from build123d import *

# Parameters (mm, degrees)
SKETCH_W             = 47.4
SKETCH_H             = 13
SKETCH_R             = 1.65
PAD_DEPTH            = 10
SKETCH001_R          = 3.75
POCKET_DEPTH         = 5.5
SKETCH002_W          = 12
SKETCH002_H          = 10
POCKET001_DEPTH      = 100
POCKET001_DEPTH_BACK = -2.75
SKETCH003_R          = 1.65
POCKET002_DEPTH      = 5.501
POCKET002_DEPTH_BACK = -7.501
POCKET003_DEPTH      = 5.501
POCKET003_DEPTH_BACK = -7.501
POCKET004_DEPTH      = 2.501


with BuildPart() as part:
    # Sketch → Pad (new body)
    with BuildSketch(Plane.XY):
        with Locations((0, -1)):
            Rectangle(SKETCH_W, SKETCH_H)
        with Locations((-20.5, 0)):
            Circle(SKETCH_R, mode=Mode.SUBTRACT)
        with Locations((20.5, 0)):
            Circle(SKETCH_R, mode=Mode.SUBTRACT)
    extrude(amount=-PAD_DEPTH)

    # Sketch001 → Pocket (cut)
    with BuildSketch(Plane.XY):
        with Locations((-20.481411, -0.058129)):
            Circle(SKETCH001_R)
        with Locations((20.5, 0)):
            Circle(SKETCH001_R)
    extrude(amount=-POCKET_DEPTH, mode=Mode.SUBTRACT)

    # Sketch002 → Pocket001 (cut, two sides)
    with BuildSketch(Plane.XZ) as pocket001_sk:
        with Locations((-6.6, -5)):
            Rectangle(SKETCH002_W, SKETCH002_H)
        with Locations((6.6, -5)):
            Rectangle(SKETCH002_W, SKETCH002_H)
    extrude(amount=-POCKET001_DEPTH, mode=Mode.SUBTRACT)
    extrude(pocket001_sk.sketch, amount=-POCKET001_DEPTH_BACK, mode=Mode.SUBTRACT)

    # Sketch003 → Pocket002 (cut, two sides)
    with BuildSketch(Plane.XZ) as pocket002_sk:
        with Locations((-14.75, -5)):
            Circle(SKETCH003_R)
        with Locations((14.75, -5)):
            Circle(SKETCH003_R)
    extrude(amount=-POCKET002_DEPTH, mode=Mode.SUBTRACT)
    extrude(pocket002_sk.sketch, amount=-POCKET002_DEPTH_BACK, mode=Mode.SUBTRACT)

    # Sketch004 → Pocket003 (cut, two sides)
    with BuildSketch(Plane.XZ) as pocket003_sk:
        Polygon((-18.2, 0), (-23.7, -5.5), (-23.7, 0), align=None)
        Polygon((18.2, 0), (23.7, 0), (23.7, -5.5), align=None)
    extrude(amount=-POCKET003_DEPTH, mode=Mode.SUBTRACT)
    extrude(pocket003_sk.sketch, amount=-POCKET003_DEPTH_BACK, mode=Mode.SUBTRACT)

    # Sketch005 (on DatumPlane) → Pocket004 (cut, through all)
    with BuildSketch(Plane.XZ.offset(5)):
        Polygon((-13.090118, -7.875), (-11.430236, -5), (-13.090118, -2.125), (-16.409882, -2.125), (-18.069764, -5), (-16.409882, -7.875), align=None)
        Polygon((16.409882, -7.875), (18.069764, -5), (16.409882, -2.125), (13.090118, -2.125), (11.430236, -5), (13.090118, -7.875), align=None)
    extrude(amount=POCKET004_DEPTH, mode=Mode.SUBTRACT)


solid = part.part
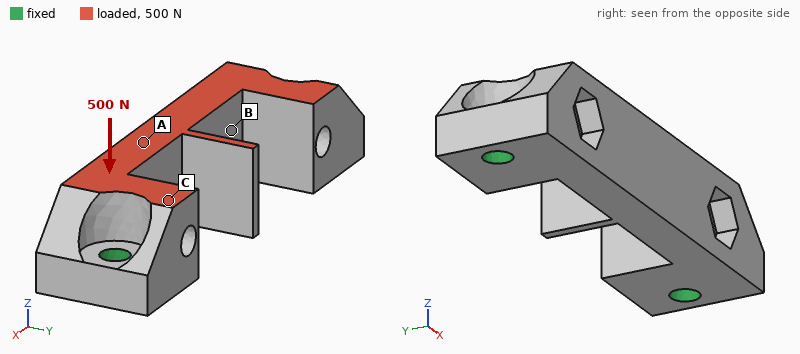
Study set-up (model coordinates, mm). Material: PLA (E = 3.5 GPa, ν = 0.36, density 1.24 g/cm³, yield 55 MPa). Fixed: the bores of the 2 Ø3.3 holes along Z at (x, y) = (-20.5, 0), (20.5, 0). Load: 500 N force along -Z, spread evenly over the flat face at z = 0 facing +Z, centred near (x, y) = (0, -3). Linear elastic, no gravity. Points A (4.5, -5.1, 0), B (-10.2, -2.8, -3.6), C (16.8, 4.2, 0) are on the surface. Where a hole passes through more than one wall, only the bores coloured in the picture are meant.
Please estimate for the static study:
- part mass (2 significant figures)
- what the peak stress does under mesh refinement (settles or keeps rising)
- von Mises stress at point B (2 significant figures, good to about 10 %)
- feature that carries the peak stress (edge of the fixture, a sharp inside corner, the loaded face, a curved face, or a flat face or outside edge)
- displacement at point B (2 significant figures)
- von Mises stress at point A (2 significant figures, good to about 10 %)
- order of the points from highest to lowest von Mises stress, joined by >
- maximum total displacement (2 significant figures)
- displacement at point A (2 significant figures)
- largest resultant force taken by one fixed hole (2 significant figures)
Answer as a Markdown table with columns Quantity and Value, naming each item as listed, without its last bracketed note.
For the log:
| Quantity | Value |
|---|---|
| part mass | 3.9 g |
| what the peak stress does under mesh refinement | keeps rising |
| von Mises stress at point B | 8.2 MPa |
| feature that carries the peak stress | edge of the fixture |
| displacement at point B | 0.14 mm |
| von Mises stress at point A | 14 MPa |
| order of the points from highest to lowest von Mises stress, joined by > | A > B > C |
| maximum total displacement | 0.22 mm |
| displacement at point A | 0.19 mm |
| largest resultant force taken by one fixed hole | 260 N |
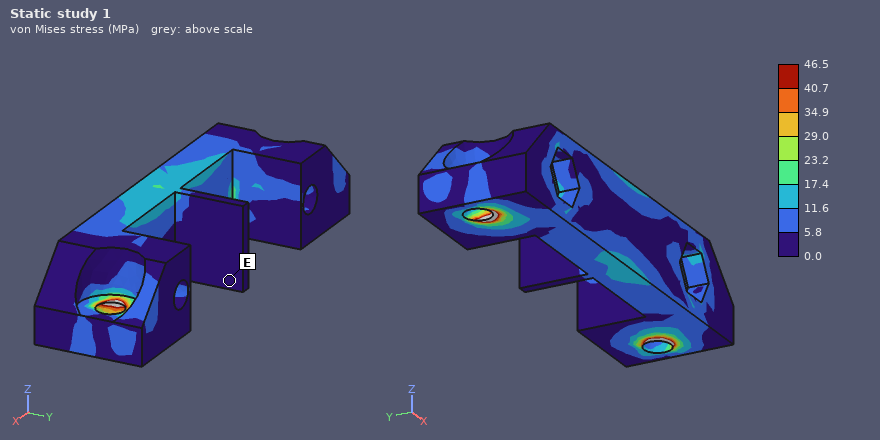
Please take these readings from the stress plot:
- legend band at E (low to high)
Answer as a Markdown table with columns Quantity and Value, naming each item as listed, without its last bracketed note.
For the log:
| Quantity | Value |
|---|---|
| legend band at E | 0.0 to 5.8 MPa |
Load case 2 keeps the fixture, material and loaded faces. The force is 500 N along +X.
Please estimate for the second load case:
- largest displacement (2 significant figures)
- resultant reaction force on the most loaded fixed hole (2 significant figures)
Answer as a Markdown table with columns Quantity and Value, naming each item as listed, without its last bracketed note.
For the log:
| Quantity | Value |
|---|---|
| largest displacement | 0.56 mm |
| resultant reaction force on the most loaded fixed hole | 260 N |
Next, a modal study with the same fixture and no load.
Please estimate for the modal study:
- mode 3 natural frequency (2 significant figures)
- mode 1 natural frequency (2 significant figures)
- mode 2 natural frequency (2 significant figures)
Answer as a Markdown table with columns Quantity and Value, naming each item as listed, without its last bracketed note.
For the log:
| Quantity | Value |
|---|---|
| mode 3 natural frequency | 6000 Hz |
| mode 1 natural frequency | 4500 Hz |
| mode 2 natural frequency | 4600 Hz |
